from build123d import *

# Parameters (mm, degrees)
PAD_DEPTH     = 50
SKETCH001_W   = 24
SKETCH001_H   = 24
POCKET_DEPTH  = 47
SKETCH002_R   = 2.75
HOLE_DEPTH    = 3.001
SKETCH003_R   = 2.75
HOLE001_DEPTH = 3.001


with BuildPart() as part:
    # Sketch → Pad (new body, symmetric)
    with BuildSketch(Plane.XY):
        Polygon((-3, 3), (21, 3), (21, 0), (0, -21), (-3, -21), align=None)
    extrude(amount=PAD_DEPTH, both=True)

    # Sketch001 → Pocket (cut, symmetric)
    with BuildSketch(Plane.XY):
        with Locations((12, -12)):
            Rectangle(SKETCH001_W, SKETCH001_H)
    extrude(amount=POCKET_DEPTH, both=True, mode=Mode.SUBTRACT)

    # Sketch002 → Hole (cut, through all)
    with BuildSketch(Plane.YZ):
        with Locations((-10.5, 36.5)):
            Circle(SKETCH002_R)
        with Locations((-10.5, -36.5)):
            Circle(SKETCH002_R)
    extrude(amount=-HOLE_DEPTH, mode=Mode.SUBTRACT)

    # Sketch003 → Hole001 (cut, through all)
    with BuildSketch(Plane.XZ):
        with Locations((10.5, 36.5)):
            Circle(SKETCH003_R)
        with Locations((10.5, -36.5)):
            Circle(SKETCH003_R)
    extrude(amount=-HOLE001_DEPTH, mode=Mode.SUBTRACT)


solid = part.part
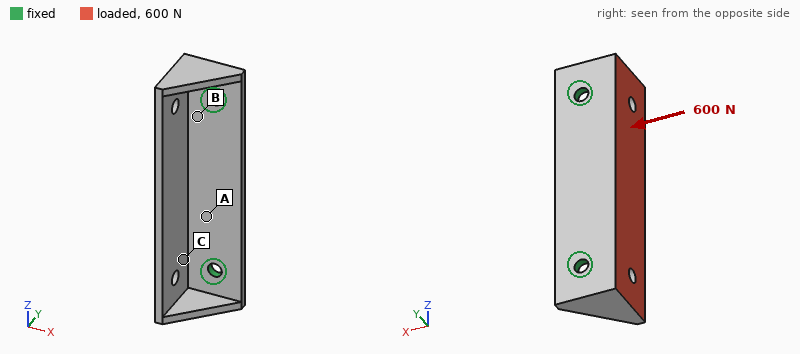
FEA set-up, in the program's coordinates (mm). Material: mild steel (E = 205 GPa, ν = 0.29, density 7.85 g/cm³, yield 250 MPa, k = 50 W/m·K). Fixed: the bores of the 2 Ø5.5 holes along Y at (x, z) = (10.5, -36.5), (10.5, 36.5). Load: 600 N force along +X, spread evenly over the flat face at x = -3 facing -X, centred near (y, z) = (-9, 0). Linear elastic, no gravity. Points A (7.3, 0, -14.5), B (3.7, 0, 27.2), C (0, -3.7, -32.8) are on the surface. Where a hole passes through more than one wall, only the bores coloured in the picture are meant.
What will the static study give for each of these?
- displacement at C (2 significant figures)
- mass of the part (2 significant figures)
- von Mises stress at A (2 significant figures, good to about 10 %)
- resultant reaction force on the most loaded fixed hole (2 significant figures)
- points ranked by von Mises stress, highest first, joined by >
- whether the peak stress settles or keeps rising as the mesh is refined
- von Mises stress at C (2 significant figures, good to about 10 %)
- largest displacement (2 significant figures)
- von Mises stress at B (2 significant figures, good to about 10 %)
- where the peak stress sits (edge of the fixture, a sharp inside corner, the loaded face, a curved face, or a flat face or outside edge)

10 µm
110 g
21 MPa
310 N
B > A > C
keeps rising
14 MPa
54 µm
32 MPa
edge of the fixture
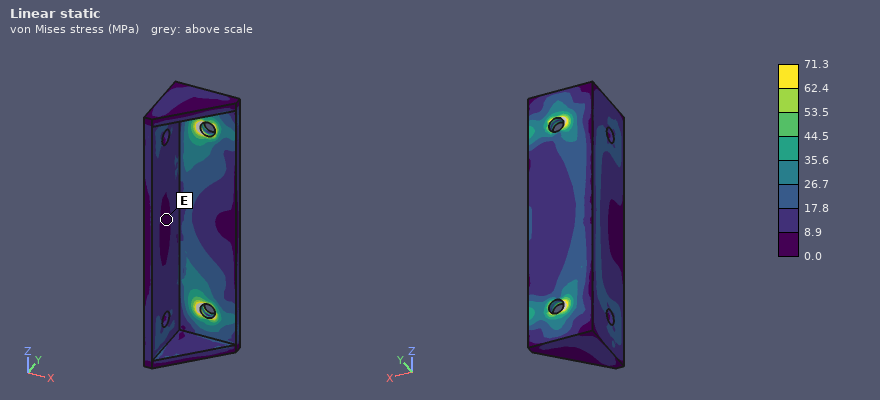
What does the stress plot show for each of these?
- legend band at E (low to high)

0.0 to 8.9 MPa
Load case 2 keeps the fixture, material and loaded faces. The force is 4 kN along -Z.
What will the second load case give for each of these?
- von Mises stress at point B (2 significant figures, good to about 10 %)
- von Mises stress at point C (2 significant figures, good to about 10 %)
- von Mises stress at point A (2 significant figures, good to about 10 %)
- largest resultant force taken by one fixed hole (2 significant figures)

61 MPa
36 MPa
32 MPa
2.2 kN
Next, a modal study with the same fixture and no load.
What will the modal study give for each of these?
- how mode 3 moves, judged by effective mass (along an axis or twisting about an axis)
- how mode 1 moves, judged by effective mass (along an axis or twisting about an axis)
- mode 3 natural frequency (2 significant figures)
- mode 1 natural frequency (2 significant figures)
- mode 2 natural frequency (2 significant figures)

along Y
along X
4500 Hz
2700 Hz
4100 Hz
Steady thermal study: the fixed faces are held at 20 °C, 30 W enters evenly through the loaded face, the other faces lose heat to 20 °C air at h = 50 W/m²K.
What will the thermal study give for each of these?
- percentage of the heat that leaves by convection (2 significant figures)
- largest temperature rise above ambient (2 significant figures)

35 %
49 K
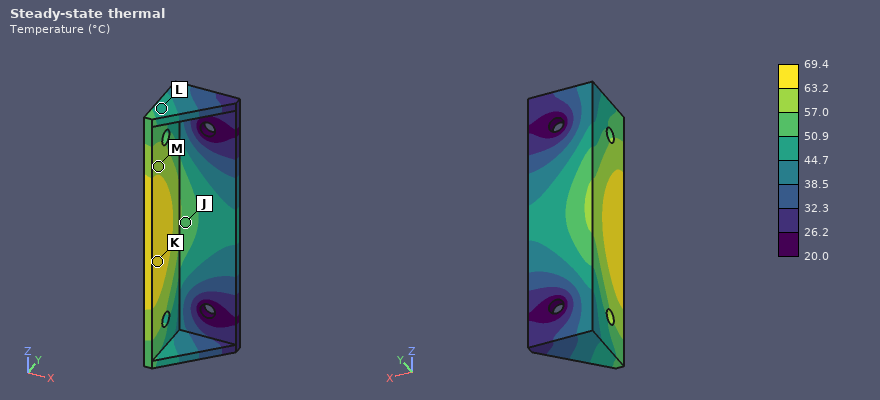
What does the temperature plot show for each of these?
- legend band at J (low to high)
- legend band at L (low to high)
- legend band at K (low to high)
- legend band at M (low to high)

50.9 to 57.0 °C
44.7 to 50.9 °C
63.2 to 69.4 °C
57.0 to 63.2 °C
